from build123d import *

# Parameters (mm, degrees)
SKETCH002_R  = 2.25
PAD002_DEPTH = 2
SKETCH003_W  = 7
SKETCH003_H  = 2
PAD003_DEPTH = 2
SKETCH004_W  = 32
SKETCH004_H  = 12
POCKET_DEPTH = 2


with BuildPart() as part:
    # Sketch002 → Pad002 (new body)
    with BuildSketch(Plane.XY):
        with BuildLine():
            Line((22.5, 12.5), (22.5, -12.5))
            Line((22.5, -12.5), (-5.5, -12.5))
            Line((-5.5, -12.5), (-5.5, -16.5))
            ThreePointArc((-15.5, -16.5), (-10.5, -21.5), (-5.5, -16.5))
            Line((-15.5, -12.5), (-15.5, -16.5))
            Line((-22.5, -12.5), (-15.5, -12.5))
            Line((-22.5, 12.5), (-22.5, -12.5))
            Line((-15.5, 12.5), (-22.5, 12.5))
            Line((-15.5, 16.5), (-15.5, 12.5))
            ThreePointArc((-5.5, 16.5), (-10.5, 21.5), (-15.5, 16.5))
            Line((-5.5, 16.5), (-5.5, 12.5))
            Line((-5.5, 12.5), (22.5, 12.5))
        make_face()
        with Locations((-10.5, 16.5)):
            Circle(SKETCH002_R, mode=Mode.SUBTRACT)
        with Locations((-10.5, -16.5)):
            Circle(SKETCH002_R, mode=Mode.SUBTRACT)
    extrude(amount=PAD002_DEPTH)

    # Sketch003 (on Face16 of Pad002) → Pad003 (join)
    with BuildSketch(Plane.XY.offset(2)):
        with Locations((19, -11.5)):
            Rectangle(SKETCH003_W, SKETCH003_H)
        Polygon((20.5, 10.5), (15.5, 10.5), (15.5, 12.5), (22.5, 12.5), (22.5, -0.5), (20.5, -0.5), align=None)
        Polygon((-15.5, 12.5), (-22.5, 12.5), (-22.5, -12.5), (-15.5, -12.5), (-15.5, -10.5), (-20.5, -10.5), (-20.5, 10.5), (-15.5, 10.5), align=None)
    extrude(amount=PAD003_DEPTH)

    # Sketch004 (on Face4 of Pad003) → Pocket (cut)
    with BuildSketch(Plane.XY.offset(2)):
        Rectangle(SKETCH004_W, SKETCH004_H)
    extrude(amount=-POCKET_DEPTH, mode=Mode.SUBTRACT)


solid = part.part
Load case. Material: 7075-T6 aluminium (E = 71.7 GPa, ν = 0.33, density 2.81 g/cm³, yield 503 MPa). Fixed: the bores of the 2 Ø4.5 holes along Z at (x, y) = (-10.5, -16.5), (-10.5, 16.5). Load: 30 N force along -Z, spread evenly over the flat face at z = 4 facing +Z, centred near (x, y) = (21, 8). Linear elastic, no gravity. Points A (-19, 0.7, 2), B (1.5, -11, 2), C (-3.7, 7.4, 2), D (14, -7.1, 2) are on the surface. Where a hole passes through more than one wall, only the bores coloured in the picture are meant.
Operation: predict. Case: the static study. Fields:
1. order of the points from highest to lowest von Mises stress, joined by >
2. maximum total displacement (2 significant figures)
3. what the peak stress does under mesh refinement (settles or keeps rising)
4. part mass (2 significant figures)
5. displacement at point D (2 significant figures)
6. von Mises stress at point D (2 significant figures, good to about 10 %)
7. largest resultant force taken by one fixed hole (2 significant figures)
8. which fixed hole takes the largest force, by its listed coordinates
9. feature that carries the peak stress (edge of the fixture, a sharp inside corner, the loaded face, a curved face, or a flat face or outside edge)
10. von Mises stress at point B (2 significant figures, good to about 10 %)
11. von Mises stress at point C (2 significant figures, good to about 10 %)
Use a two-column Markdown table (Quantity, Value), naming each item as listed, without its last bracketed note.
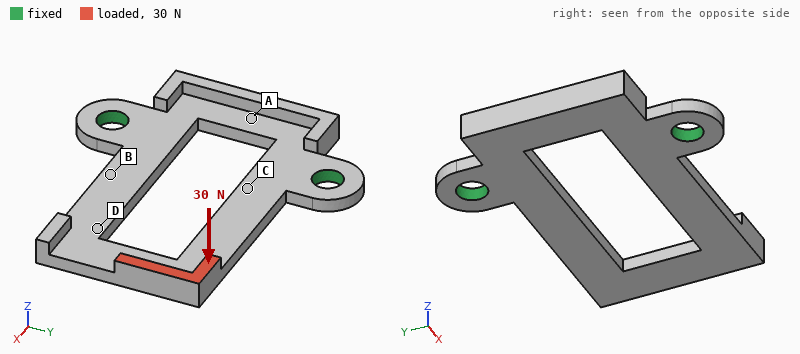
| Quantity | Value |
|---|---|
| order of the points from highest to lowest von Mises stress, joined by > | C > B > D > A |
| maximum total displacement | 0.57 mm |
| what the peak stress does under mesh refinement | keeps rising |
| part mass | 5.6 g |
| displacement at point D | 0.29 mm |
| von Mises stress at point D | 33 MPa |
| largest resultant force taken by one fixed hole | 22 N |
| which fixed hole takes the largest force, by its listed coordinates | (-10.5, 16.5) |
| feature that carries the peak stress | a sharp inside corner |
| von Mises stress at point B | 60 MPa |
| von Mises stress at point C | 90 MPa |
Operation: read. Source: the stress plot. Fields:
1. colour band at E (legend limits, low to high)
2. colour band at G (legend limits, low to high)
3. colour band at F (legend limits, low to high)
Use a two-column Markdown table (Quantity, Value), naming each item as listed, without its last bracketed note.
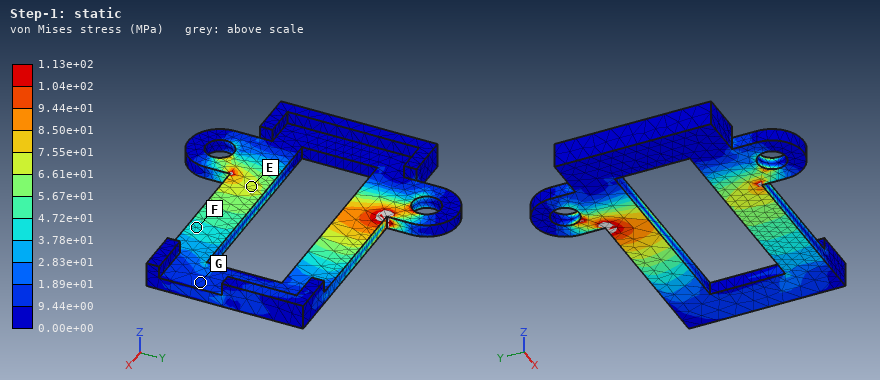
| Quantity | Value |
|---|---|
| colour band at E | 6.61e+01 to 7.55e+01 MPa |
| colour band at G | 9.44e+00 to 1.89e+01 MPa |
| colour band at F | 3.78e+01 to 4.72e+01 MPa |
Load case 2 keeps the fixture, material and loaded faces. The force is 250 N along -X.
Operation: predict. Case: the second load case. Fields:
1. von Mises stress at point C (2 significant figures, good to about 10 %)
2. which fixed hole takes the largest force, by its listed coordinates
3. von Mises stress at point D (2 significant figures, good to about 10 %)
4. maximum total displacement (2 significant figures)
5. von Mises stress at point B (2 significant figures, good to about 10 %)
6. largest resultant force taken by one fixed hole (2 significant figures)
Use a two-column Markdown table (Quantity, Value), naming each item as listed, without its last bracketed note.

| Quantity | Value |
|---|---|
| von Mises stress at point C | 95 MPa |
| which fixed hole takes the largest force, by its listed coordinates | (-10.5, 16.5) |
| von Mises stress at point D | 80 MPa |
| maximum total displacement | 0.69 mm |
| von Mises stress at point B | 81 MPa |
| largest resultant force taken by one fixed hole | 210 N |
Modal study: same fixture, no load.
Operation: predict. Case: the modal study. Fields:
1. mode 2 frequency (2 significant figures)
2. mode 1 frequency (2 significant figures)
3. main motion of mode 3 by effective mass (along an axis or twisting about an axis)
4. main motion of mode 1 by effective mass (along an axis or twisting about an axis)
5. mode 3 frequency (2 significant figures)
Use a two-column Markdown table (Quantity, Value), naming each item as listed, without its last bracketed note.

| Quantity | Value |
|---|---|
| mode 2 frequency | 3300 Hz |
| mode 1 frequency | 1100 Hz |
| main motion of mode 3 by effective mass | along Z |
| main motion of mode 1 by effective mass | along Z |
| mode 3 frequency | 6300 Hz |
